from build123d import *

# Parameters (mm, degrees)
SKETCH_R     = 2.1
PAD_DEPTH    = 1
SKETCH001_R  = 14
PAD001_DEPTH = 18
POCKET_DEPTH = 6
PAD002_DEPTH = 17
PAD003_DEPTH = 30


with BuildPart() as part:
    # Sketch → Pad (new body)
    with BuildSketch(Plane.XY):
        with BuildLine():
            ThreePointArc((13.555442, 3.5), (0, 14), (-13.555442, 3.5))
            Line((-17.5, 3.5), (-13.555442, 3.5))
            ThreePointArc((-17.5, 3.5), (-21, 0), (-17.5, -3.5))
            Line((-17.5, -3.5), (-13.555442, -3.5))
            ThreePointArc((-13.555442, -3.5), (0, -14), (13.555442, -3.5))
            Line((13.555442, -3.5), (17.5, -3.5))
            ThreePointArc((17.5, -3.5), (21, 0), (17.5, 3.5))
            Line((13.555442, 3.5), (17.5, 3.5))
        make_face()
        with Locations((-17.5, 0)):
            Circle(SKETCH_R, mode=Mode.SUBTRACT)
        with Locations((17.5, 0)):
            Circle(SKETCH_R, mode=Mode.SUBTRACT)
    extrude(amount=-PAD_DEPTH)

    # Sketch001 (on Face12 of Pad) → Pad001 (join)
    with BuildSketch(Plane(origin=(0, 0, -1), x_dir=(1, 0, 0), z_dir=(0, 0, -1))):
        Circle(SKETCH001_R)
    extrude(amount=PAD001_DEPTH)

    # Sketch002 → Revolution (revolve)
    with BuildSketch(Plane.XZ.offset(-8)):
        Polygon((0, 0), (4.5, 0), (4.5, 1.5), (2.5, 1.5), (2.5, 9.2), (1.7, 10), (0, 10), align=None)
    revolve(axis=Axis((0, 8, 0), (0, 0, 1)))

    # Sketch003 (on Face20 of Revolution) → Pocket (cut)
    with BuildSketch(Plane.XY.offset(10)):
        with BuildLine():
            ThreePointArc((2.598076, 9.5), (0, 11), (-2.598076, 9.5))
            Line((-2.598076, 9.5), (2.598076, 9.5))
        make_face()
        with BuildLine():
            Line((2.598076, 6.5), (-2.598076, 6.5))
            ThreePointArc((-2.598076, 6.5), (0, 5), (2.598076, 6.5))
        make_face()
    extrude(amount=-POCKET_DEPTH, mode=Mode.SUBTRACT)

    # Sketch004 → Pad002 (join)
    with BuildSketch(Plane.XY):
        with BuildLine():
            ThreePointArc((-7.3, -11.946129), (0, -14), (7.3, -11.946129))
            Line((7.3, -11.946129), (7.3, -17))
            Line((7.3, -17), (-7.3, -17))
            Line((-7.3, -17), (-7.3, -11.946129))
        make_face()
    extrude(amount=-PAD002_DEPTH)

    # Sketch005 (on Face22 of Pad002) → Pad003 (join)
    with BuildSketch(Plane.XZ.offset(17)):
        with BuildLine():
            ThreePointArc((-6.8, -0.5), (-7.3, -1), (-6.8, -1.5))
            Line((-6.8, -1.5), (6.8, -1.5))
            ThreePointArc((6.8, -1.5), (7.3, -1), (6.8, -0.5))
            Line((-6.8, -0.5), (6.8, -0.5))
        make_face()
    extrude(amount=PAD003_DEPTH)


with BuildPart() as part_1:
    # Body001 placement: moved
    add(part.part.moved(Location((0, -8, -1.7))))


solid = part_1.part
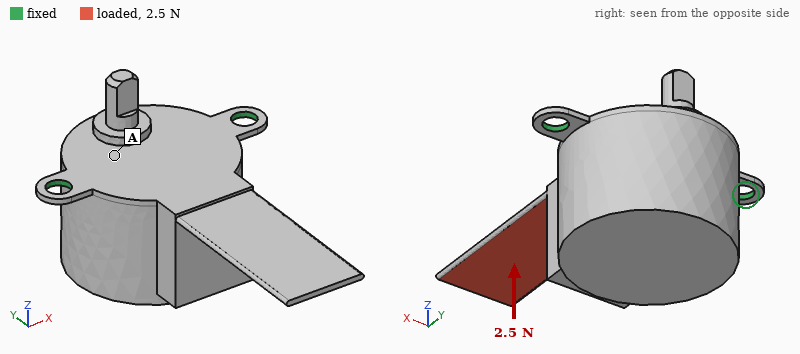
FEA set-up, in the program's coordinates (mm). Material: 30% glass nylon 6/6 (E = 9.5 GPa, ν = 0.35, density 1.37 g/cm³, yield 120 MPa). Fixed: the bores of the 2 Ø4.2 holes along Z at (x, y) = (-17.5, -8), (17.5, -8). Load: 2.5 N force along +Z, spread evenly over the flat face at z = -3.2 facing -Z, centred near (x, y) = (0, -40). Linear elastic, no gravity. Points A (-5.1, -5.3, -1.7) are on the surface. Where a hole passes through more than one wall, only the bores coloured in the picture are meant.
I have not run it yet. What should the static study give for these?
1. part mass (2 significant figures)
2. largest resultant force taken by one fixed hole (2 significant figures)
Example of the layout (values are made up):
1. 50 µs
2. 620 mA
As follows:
1. 18 g
2. 1.6 N
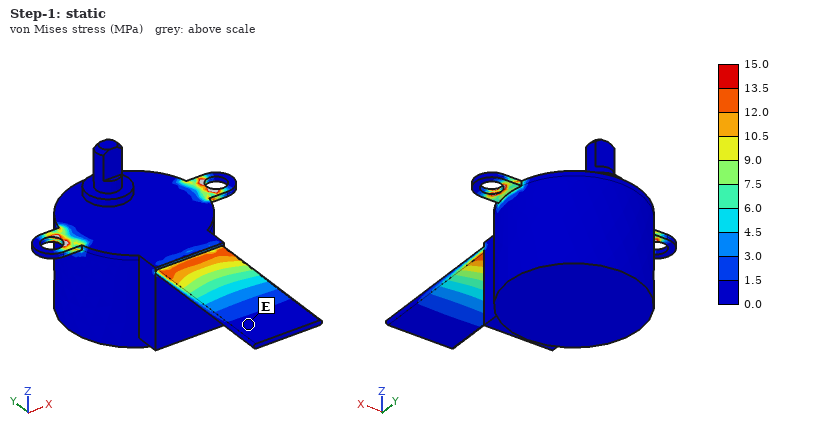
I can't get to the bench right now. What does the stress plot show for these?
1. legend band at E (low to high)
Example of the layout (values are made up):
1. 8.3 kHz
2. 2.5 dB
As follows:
1. 0.0 to 1.5 MPa
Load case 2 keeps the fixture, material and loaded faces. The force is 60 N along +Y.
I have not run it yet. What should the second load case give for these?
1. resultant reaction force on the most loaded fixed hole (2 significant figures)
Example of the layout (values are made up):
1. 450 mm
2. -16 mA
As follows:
1. 30 N
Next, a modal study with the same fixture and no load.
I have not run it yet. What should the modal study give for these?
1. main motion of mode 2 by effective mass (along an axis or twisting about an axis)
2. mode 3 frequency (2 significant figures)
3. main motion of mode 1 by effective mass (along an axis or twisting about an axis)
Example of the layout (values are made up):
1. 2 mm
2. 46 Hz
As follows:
1. along Y
2. 2000 Hz
3. along Y
